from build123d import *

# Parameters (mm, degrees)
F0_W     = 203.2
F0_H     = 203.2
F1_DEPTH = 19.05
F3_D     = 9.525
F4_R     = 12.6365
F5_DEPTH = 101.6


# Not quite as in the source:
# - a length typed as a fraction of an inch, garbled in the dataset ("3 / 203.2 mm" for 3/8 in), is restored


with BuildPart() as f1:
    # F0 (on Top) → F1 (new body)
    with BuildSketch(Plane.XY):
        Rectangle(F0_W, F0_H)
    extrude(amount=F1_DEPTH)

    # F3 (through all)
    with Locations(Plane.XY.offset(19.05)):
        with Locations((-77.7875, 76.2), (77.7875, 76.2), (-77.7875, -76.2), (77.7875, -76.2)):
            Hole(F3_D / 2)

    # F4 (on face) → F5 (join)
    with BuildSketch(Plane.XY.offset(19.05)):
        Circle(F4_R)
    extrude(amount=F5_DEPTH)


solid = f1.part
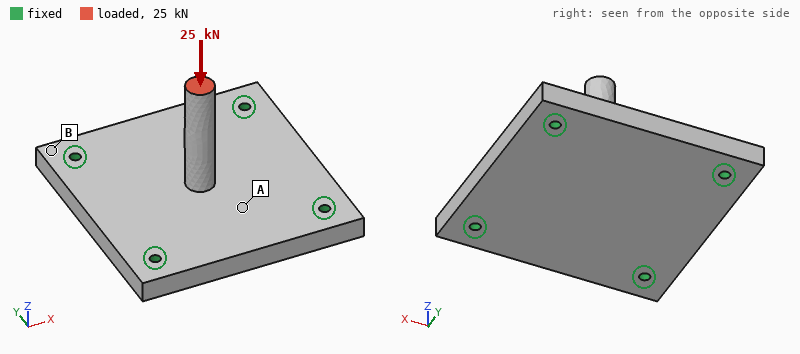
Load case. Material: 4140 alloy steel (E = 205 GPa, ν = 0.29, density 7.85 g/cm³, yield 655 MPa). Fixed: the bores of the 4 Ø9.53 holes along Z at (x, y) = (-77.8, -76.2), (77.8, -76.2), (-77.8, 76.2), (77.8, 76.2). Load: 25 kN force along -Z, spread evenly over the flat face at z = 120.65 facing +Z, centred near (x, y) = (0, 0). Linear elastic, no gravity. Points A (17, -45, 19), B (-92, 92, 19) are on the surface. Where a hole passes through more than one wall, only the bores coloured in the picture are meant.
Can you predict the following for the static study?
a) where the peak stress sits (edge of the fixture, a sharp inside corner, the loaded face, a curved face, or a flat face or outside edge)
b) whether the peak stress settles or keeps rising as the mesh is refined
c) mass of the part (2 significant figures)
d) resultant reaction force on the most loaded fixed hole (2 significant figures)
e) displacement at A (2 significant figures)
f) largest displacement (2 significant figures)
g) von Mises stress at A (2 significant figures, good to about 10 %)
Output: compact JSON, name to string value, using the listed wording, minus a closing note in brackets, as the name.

{"where the peak stress sits": "edge of the fixture", "whether the peak stress settles or keeps rising as the mesh is refined": "keeps rising", "mass of the part": "6.5 kg", "resultant reaction force on the most loaded fixed hole": "6.3 kN", "displacement at A": "45 µm", "largest displacement": "96 µm", "von Mises stress at A": "30 MPa"}
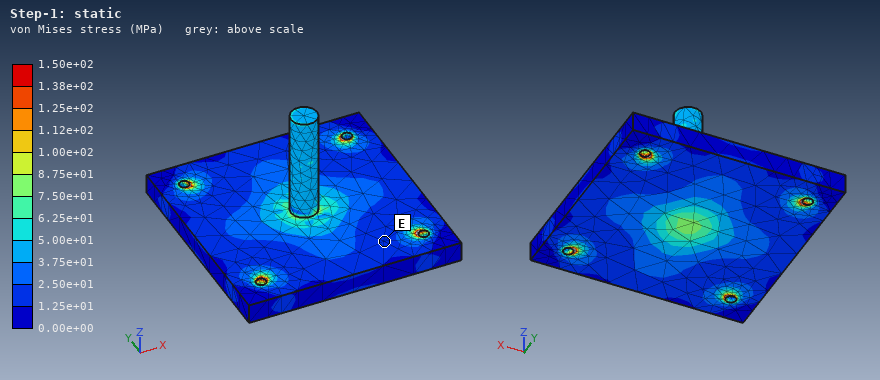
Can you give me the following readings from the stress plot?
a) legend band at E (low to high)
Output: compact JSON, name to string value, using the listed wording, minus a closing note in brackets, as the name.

{"legend band at E": "1.25e+01 to 2.50e+01 MPa"}
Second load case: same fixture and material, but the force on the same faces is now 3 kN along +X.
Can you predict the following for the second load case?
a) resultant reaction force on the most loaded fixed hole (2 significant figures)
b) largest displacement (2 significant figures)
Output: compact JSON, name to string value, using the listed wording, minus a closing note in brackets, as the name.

{"resultant reaction force on the most loaded fixed hole": "1.5 kN", "largest displacement": "0.35 mm"}
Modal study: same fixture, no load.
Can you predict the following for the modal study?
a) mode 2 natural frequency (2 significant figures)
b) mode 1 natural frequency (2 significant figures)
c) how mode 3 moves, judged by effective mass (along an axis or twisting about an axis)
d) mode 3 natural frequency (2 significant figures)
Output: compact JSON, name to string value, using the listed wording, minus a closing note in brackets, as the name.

{"mode 2 natural frequency": "1400 Hz", "mode 1 natural frequency": "1400 Hz", "how mode 3 moves, judged by effective mass": "along Z", "mode 3 natural frequency": "2200 Hz"}
